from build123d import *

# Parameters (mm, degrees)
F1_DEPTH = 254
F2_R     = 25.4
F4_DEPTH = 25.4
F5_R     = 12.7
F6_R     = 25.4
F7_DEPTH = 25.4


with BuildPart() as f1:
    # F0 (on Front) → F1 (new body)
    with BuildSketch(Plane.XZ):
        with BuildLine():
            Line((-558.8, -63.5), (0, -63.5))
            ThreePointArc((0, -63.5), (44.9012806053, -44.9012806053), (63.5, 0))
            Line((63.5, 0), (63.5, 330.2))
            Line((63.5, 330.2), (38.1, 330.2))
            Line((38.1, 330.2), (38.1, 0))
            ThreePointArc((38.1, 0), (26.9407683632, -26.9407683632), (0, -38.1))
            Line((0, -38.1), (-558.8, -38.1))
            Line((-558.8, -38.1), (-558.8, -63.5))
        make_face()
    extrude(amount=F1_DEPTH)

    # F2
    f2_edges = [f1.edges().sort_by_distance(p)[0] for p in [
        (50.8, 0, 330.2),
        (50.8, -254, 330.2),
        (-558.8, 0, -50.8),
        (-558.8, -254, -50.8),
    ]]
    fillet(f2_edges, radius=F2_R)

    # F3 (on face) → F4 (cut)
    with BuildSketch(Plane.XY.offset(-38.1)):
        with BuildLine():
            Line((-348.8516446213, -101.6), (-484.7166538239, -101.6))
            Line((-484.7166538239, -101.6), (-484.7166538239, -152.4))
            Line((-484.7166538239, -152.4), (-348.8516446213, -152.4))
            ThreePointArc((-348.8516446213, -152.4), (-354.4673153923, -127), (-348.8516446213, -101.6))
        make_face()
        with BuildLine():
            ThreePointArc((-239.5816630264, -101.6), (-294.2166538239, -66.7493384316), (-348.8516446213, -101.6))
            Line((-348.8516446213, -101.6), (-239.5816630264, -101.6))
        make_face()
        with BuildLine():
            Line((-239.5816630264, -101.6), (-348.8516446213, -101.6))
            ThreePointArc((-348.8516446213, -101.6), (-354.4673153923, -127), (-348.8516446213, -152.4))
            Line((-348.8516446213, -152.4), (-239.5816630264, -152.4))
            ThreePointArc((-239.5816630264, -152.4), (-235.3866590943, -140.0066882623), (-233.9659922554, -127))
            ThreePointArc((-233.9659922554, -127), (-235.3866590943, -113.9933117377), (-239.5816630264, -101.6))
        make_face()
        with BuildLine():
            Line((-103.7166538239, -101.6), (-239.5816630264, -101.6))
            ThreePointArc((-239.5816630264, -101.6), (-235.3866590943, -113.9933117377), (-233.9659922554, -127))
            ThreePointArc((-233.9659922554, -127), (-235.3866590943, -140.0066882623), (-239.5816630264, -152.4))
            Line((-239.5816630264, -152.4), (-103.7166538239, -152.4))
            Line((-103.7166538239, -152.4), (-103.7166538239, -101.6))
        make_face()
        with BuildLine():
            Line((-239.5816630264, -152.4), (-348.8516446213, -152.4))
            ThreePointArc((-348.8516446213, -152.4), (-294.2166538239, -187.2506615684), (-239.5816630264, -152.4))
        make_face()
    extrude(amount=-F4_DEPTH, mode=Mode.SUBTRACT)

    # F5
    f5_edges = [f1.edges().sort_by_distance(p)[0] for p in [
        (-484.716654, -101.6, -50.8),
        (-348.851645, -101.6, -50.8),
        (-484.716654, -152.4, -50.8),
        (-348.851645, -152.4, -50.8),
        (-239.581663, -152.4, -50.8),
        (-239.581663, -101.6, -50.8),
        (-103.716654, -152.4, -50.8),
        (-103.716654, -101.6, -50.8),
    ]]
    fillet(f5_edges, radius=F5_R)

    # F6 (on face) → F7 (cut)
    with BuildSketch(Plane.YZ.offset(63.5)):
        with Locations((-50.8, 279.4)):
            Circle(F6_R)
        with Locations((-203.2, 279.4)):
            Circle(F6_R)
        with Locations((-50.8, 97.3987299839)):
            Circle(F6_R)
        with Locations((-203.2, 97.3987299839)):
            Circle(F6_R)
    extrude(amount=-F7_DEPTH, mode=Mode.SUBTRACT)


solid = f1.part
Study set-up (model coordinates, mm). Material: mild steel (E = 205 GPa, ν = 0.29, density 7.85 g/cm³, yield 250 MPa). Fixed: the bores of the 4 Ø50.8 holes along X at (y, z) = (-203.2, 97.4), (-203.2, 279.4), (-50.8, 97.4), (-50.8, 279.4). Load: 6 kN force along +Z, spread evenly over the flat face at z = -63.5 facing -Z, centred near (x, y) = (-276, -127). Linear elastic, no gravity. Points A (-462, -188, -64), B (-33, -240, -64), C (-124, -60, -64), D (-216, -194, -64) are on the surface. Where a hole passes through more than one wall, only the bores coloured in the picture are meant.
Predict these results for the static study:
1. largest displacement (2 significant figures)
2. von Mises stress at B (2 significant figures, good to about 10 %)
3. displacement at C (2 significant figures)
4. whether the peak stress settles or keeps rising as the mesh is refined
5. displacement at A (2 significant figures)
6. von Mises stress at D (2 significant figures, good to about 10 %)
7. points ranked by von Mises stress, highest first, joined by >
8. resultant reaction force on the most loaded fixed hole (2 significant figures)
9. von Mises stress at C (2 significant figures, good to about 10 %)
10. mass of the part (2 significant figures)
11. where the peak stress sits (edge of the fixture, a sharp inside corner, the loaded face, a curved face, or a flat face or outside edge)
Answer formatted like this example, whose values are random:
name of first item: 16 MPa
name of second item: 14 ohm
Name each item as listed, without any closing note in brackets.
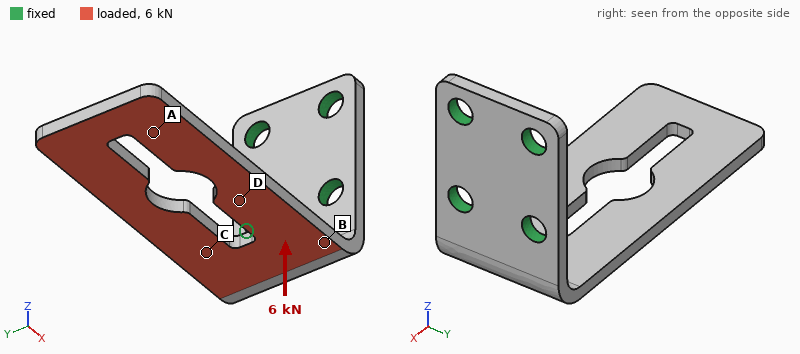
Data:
largest displacement: 4.6 mm
von Mises stress at B: 57 MPa
displacement at C: 0.89 mm
whether the peak stress settles or keeps rising as the mesh is refined: keeps rising
displacement at A: 3.7 mm
von Mises stress at D: 31 MPa
points ranked by von Mises stress, highest first, joined by >: B > C > D > A
resultant reaction force on the most loaded fixed hole: 3.5 kN
von Mises stress at C: 45 MPa
mass of the part: 42 kg
where the peak stress sits: edge of the fixture
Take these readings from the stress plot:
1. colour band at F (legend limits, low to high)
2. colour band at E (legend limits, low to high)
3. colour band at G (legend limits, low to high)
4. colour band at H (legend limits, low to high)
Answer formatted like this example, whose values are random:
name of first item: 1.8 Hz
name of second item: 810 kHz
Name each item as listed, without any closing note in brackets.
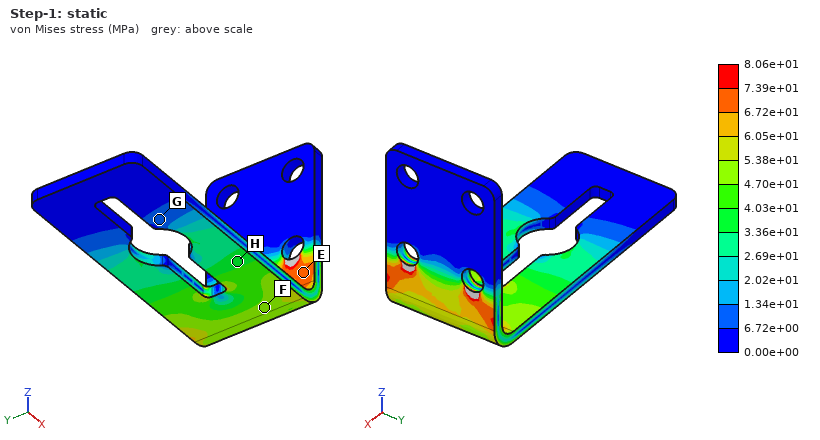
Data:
colour band at F: 4.70e+01 to 5.38e+01 MPa
colour band at E: 6.72e+01 to 7.39e+01 MPa
colour band at G: 6.72e+00 to 1.34e+01 MPa
colour band at H: 3.36e+01 to 4.03e+01 MPa
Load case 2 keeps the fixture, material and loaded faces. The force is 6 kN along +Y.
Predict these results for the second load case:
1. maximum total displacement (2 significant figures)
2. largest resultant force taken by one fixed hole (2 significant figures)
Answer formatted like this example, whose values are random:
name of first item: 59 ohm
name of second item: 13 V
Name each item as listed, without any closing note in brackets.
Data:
maximum total displacement: 0.65 mm
largest resultant force taken by one fixed hole: 12 kN
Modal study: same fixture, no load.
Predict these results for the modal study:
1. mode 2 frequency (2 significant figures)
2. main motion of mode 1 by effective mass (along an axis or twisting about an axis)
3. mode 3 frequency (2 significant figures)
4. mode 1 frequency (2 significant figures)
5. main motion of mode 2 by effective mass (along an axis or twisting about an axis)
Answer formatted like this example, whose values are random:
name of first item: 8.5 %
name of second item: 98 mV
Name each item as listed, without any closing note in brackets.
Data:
mode 2 frequency: 120 Hz
main motion of mode 1 by effective mass: along Z
mode 3 frequency: 240 Hz
mode 1 frequency: 46 Hz
main motion of mode 2 by effective mass: along Y
